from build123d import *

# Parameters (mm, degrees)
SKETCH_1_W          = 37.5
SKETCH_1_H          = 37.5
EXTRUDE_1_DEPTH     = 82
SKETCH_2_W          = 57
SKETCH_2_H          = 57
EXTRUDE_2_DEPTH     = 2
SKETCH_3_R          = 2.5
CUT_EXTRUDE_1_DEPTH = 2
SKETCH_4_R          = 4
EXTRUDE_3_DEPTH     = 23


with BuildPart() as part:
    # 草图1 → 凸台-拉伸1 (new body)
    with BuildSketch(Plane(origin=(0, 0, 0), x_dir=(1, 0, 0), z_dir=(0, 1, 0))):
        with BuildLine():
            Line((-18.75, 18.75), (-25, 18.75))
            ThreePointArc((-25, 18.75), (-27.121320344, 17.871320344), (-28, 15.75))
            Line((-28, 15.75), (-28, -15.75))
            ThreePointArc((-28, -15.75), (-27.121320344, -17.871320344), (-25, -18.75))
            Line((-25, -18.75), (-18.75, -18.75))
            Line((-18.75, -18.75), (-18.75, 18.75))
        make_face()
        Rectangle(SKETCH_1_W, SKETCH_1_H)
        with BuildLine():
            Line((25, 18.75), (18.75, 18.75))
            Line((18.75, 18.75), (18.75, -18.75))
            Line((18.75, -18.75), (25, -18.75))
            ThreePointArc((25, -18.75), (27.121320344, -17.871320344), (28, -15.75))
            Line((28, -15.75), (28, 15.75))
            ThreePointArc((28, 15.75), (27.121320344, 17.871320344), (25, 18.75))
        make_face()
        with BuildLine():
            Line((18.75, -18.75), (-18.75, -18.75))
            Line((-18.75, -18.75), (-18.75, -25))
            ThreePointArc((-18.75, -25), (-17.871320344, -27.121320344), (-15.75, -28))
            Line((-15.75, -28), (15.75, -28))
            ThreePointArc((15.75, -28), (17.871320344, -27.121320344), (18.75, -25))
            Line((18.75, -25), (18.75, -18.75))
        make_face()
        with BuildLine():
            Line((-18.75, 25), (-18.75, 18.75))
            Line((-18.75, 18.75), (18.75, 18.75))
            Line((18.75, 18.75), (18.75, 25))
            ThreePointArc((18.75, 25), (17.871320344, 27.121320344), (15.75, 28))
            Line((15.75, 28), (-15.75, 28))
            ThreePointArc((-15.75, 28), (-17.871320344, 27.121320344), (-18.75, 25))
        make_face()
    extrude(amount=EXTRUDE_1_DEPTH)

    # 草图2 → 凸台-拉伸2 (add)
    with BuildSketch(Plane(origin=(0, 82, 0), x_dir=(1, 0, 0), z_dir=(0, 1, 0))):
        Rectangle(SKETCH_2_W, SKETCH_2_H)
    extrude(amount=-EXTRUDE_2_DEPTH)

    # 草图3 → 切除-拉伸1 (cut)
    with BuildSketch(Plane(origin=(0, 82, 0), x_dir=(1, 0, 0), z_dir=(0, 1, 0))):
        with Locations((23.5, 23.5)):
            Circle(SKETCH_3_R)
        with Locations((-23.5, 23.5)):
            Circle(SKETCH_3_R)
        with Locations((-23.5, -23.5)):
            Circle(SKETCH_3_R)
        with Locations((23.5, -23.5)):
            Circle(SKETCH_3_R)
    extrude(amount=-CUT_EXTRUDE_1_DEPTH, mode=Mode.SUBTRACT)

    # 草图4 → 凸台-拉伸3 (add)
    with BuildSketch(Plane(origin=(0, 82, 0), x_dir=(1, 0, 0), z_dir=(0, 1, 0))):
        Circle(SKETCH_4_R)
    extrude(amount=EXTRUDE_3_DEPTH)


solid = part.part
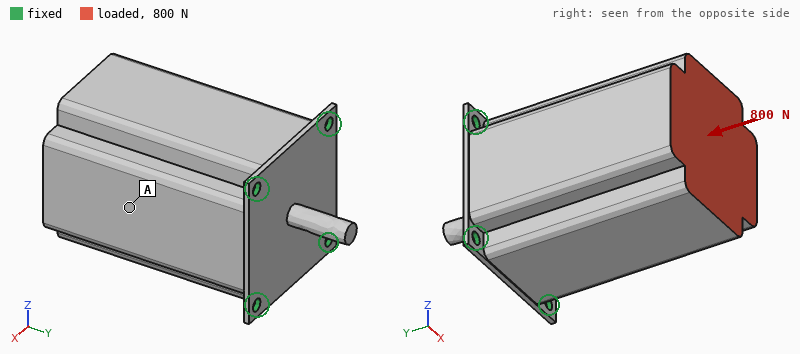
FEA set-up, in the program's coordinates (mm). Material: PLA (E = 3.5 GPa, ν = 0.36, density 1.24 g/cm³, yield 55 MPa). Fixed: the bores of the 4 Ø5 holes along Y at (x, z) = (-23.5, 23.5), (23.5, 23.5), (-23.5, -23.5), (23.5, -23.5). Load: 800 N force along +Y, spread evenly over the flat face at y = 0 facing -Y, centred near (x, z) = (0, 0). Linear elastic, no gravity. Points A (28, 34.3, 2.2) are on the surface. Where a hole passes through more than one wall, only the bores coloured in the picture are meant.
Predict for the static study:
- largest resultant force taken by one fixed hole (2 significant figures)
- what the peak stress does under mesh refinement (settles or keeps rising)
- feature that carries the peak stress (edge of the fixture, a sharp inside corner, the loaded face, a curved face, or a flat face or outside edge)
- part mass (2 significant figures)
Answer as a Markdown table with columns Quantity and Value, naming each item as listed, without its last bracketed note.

| Quantity | Value |
|---|---|
| largest resultant force taken by one fixed hole | 220 N |
| what the peak stress does under mesh refinement | keeps rising |
| feature that carries the peak stress | edge of the fixture |
| part mass | 280 g |
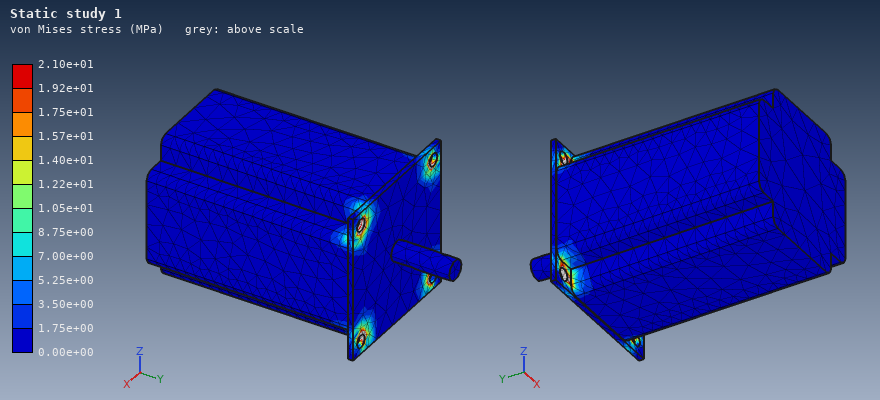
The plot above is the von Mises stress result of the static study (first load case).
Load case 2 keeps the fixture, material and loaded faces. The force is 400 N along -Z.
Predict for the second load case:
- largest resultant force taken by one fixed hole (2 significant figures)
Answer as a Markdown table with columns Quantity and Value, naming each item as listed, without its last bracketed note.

| Quantity | Value |
|---|---|
| largest resultant force taken by one fixed hole | 410 N |
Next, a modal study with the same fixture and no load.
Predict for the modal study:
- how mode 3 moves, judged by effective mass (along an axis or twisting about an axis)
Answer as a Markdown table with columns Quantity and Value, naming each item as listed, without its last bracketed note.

| Quantity | Value |
|---|---|
| how mode 3 moves, judged by effective mass | along Y |
